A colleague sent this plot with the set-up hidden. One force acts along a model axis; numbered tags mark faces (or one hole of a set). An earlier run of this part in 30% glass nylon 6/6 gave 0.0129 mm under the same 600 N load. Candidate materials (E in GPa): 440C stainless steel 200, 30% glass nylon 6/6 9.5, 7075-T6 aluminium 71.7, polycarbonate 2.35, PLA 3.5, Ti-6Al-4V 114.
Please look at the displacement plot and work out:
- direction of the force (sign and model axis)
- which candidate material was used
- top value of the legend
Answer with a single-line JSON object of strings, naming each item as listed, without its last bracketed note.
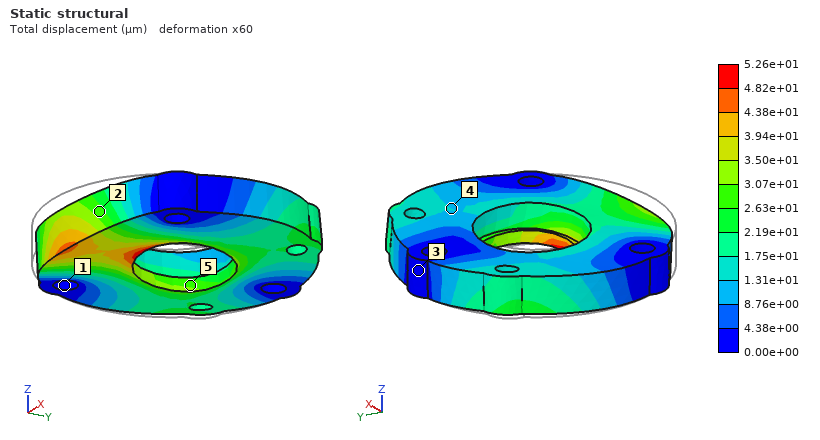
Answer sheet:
{"direction of the force": "+Y", "which candidate material was used": "polycarbonate", "top value of the legend": "5.26e+01 µm"}
